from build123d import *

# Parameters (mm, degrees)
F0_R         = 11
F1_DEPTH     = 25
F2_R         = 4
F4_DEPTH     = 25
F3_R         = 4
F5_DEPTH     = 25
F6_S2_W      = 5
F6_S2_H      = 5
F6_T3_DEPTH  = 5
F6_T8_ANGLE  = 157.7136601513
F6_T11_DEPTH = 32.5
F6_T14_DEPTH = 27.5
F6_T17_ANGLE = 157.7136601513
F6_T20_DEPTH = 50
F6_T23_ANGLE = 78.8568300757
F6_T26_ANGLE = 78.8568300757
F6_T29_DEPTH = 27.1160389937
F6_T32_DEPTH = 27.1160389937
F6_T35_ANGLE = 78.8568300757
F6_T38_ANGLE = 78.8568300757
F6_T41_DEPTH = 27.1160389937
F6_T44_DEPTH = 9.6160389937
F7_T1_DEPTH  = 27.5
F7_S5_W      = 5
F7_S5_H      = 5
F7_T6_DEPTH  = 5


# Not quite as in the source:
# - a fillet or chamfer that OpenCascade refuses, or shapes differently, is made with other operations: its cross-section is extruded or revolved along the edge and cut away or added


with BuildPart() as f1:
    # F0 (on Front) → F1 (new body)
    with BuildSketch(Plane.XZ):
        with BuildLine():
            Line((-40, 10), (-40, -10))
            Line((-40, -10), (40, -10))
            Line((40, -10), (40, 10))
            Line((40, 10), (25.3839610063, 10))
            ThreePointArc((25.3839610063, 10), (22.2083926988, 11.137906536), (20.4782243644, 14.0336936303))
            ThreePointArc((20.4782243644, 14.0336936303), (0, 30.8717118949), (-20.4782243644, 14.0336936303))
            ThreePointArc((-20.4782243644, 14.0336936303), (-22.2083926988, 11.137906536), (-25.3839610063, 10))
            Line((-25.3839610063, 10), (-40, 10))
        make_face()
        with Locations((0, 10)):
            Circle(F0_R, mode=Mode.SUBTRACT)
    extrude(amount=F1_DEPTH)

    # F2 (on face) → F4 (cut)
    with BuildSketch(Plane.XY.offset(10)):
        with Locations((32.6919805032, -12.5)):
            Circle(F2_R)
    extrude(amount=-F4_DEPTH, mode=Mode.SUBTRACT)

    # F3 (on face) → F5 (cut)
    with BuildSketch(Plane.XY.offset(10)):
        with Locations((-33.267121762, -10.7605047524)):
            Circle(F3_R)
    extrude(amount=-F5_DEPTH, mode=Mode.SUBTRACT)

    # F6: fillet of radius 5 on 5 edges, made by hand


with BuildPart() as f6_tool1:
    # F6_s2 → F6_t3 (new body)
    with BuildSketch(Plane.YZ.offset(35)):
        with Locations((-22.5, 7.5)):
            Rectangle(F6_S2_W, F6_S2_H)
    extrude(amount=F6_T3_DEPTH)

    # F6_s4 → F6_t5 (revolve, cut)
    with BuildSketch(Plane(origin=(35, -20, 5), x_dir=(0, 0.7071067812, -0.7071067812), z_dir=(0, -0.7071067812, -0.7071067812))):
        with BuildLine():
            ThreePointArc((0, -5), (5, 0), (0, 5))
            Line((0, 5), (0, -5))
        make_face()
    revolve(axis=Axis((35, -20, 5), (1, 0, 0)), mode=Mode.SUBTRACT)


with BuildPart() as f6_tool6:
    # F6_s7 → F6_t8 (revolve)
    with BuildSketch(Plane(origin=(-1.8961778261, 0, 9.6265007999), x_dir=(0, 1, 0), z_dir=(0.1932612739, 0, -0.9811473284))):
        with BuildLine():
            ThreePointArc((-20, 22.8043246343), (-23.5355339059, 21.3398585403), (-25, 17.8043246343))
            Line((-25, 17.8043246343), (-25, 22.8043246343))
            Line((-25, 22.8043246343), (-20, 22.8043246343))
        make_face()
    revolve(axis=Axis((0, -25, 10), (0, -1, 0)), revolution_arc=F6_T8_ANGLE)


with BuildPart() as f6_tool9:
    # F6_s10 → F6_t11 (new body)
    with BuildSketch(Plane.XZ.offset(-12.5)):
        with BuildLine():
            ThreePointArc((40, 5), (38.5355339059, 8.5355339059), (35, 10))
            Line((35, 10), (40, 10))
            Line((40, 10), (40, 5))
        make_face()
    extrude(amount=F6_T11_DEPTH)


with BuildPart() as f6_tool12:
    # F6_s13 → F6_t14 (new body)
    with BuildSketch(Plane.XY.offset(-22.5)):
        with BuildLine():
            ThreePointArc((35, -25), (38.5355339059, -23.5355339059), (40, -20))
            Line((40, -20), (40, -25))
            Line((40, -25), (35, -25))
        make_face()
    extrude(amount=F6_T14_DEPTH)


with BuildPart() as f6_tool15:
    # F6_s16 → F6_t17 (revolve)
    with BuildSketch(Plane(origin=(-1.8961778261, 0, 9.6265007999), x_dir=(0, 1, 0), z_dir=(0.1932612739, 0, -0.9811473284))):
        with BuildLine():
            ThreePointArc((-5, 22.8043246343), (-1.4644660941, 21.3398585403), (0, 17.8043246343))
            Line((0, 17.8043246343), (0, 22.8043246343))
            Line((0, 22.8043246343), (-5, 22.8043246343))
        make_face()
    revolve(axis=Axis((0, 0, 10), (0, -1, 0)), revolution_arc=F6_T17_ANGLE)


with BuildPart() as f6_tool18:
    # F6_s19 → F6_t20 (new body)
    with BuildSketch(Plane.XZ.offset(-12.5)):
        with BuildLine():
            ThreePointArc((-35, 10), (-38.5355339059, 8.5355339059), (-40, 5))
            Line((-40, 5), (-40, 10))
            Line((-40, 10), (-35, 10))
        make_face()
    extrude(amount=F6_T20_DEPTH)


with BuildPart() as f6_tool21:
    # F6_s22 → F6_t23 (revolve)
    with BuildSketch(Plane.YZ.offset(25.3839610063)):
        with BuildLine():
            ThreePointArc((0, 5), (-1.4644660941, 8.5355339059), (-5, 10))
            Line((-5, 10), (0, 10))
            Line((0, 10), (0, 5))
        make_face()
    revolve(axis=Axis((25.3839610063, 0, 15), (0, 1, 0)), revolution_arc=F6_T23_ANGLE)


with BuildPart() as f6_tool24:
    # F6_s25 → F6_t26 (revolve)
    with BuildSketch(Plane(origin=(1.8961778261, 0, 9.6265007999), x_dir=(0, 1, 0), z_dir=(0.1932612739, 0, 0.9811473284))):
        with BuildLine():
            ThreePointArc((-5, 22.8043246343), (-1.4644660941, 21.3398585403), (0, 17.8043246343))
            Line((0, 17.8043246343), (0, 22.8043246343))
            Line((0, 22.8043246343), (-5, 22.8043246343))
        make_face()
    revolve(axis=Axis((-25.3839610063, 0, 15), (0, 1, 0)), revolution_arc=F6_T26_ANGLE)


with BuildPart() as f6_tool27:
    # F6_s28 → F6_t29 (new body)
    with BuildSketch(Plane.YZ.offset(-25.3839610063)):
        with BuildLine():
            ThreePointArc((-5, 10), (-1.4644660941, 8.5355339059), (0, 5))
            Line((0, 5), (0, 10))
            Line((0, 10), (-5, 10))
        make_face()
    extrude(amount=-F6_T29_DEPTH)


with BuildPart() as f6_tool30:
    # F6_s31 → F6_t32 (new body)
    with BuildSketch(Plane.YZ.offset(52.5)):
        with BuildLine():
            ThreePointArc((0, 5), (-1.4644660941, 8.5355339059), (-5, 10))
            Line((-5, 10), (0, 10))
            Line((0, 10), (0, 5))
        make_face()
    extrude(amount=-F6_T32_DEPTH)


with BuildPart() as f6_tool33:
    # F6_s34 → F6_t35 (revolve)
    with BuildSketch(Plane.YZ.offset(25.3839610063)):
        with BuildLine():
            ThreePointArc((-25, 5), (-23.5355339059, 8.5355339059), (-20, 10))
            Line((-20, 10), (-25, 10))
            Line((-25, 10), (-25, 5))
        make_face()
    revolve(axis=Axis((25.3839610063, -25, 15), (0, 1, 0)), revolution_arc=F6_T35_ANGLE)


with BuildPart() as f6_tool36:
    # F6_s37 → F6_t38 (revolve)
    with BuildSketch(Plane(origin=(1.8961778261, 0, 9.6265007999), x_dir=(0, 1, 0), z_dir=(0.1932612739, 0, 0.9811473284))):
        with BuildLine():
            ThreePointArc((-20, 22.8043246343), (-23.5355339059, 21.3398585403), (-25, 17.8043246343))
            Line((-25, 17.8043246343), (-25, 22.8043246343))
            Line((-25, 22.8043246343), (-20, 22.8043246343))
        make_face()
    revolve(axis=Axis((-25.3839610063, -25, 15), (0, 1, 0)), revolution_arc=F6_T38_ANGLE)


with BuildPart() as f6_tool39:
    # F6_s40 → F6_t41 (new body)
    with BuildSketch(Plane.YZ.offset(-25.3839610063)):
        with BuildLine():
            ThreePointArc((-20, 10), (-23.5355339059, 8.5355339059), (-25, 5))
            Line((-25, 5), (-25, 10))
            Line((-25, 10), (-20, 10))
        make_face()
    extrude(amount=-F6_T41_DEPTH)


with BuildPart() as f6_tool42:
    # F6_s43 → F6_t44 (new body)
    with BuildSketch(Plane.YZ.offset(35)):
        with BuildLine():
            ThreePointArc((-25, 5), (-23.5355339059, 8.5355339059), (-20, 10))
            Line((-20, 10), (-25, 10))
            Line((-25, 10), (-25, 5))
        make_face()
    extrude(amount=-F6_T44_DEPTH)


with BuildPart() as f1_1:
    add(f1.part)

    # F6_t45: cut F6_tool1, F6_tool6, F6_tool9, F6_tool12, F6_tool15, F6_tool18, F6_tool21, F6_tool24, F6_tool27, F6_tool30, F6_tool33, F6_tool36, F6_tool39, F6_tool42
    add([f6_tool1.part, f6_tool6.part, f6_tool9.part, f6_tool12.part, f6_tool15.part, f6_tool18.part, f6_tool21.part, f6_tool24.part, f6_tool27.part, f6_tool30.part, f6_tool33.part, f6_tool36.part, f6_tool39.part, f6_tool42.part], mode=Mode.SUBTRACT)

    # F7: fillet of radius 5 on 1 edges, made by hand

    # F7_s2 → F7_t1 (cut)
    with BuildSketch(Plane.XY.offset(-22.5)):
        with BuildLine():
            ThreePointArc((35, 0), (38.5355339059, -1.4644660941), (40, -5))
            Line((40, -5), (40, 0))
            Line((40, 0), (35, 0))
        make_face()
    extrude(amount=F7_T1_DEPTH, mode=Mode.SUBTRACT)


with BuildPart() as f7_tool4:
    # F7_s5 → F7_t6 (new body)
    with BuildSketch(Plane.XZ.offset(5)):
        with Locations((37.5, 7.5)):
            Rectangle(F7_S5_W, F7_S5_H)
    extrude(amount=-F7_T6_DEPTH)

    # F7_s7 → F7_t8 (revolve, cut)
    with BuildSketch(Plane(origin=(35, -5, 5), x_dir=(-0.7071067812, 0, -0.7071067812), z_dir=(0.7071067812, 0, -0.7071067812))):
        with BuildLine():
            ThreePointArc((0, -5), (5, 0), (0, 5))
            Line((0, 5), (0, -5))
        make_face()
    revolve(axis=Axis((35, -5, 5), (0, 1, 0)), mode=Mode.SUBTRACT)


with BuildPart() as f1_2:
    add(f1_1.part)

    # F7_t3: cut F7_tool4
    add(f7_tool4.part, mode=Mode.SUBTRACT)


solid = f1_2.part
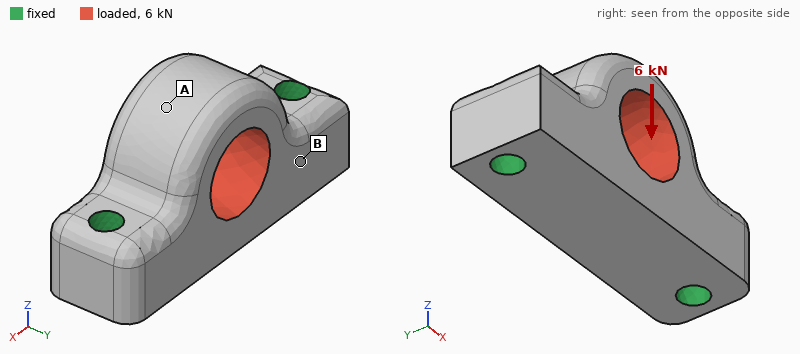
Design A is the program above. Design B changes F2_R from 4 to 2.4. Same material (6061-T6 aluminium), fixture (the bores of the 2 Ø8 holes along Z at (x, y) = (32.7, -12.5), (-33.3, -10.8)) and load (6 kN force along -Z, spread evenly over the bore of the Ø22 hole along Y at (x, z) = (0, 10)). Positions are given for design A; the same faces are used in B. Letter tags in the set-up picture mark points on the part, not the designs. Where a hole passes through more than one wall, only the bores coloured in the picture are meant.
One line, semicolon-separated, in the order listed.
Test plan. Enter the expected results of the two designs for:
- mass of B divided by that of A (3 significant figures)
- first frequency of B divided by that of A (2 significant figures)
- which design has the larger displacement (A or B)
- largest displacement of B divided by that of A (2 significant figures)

1.01; 0.94; B; 1.1
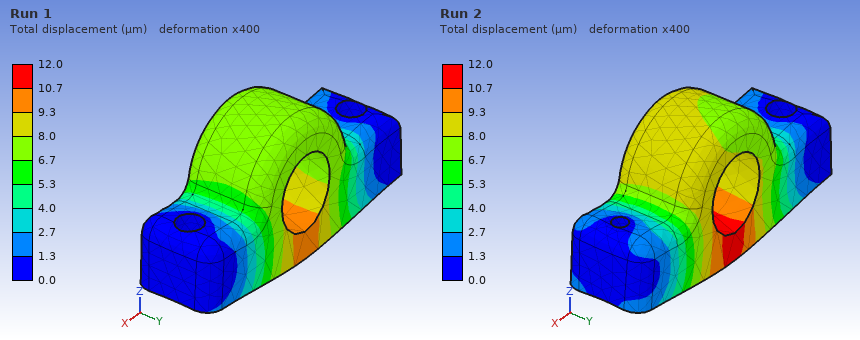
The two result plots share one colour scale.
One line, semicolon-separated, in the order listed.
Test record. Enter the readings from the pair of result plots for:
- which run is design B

Run 2
